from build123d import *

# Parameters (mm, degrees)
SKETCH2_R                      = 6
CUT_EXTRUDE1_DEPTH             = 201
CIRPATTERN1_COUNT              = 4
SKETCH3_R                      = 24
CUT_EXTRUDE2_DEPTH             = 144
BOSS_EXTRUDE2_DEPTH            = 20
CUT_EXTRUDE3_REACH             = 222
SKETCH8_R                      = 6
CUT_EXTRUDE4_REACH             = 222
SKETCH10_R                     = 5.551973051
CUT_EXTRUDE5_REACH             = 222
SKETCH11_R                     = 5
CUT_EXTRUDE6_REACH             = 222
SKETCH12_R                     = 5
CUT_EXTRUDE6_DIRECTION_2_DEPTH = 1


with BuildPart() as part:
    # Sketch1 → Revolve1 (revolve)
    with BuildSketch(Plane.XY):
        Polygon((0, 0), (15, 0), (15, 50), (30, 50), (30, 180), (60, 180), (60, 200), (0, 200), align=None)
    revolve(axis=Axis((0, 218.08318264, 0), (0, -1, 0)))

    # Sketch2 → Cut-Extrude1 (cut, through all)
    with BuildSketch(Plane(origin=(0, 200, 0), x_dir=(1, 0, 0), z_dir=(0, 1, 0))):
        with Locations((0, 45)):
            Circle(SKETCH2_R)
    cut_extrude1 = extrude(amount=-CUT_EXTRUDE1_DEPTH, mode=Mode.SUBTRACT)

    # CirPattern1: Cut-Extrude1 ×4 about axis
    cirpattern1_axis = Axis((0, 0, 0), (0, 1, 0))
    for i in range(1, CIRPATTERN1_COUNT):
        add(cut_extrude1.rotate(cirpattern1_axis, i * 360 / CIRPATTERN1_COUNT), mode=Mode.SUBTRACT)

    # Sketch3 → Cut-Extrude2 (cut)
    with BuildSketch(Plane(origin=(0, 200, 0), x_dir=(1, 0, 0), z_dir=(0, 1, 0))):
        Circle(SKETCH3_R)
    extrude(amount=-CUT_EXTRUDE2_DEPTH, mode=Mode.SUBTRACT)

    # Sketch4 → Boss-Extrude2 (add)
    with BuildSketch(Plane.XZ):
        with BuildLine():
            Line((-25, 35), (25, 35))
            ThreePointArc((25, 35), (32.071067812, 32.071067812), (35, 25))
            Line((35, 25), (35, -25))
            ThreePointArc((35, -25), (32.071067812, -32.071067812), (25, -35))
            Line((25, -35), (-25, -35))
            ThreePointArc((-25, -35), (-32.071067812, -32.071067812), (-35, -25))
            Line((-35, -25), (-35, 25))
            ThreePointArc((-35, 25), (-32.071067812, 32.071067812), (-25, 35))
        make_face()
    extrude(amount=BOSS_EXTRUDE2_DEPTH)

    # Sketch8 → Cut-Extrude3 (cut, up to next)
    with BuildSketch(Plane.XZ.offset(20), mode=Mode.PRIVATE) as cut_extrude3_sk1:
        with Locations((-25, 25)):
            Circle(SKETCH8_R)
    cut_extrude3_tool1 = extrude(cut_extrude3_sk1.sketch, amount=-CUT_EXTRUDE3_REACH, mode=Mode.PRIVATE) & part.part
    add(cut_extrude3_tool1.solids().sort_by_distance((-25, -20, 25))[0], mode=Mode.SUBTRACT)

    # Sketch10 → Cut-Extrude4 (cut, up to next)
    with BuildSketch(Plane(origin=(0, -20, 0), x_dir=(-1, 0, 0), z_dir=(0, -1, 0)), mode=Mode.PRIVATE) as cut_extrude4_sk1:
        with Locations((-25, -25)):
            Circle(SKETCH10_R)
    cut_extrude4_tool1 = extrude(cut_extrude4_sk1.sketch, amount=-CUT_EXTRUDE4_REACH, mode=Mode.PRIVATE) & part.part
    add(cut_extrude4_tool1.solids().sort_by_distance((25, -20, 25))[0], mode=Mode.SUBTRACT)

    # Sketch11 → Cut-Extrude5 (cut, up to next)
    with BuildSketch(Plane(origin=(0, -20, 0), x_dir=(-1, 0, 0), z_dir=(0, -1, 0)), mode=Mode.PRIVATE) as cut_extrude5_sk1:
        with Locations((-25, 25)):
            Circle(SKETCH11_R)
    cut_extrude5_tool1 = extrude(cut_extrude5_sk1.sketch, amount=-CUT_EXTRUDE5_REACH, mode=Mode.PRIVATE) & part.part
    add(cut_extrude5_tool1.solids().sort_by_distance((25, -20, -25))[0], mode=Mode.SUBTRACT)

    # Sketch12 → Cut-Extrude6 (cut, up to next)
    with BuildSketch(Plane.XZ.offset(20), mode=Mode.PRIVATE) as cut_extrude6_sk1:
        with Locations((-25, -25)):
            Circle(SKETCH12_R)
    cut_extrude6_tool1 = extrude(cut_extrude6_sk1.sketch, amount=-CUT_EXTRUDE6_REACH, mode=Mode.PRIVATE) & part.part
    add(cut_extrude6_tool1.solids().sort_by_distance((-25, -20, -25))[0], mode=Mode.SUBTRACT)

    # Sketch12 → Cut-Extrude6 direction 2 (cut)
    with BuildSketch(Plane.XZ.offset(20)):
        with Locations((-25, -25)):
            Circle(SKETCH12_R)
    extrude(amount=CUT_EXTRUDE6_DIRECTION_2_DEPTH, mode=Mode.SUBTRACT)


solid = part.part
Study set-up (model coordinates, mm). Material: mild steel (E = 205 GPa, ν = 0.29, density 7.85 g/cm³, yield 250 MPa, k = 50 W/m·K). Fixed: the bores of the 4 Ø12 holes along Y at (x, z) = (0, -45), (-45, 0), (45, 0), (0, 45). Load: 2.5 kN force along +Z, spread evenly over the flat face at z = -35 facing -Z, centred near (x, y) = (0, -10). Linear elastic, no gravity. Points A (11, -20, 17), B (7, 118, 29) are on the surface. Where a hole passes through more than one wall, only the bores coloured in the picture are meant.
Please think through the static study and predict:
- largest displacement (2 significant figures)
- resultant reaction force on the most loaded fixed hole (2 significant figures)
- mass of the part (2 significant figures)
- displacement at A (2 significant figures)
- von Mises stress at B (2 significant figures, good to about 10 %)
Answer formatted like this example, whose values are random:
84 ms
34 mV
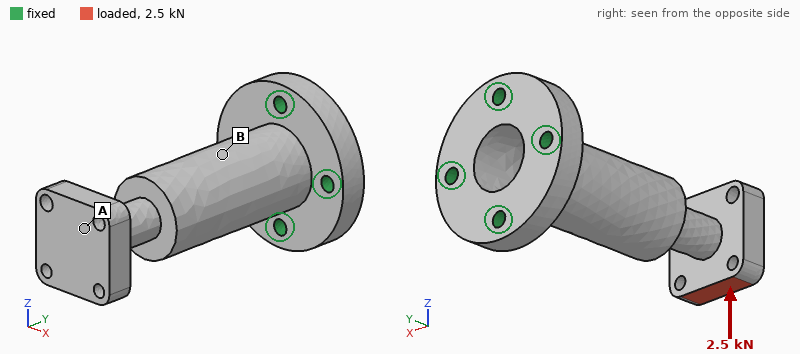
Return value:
0.19 mm
6.5 kN
3.5 kg
0.18 mm
25 MPa
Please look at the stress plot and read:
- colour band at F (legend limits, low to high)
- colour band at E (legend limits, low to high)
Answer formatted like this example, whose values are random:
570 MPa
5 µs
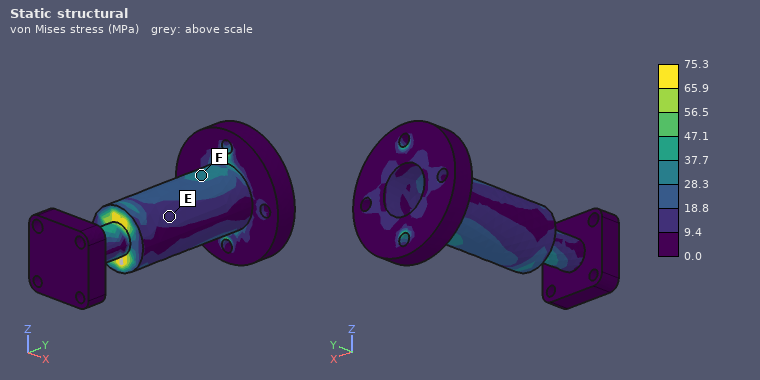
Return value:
28.3 to 37.7 MPa
9.4 to 18.8 MPa
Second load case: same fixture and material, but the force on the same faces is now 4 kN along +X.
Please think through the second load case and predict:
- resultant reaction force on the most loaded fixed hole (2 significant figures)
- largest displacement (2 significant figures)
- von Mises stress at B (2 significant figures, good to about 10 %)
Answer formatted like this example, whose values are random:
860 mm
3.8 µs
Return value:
10 kN
0.35 mm
9.8 MPa
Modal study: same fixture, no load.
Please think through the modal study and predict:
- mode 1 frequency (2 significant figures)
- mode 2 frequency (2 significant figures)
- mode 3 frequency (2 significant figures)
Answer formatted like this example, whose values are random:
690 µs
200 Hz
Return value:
660 Hz
660 Hz
2000 Hz
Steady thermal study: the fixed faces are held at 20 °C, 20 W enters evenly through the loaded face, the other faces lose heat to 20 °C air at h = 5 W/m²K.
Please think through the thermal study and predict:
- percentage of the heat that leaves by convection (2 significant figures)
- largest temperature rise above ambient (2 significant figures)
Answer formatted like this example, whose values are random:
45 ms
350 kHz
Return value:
49 %
70 K
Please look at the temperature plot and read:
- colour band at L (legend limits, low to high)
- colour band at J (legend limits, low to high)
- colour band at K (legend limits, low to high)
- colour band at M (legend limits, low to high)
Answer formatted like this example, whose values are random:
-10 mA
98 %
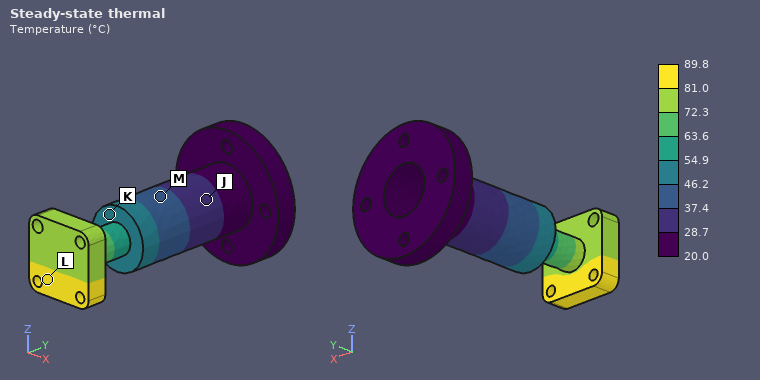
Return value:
81.0 to 89.8 °C
28.7 to 37.4 °C
46.2 to 54.9 °C
37.4 to 46.2 °C
